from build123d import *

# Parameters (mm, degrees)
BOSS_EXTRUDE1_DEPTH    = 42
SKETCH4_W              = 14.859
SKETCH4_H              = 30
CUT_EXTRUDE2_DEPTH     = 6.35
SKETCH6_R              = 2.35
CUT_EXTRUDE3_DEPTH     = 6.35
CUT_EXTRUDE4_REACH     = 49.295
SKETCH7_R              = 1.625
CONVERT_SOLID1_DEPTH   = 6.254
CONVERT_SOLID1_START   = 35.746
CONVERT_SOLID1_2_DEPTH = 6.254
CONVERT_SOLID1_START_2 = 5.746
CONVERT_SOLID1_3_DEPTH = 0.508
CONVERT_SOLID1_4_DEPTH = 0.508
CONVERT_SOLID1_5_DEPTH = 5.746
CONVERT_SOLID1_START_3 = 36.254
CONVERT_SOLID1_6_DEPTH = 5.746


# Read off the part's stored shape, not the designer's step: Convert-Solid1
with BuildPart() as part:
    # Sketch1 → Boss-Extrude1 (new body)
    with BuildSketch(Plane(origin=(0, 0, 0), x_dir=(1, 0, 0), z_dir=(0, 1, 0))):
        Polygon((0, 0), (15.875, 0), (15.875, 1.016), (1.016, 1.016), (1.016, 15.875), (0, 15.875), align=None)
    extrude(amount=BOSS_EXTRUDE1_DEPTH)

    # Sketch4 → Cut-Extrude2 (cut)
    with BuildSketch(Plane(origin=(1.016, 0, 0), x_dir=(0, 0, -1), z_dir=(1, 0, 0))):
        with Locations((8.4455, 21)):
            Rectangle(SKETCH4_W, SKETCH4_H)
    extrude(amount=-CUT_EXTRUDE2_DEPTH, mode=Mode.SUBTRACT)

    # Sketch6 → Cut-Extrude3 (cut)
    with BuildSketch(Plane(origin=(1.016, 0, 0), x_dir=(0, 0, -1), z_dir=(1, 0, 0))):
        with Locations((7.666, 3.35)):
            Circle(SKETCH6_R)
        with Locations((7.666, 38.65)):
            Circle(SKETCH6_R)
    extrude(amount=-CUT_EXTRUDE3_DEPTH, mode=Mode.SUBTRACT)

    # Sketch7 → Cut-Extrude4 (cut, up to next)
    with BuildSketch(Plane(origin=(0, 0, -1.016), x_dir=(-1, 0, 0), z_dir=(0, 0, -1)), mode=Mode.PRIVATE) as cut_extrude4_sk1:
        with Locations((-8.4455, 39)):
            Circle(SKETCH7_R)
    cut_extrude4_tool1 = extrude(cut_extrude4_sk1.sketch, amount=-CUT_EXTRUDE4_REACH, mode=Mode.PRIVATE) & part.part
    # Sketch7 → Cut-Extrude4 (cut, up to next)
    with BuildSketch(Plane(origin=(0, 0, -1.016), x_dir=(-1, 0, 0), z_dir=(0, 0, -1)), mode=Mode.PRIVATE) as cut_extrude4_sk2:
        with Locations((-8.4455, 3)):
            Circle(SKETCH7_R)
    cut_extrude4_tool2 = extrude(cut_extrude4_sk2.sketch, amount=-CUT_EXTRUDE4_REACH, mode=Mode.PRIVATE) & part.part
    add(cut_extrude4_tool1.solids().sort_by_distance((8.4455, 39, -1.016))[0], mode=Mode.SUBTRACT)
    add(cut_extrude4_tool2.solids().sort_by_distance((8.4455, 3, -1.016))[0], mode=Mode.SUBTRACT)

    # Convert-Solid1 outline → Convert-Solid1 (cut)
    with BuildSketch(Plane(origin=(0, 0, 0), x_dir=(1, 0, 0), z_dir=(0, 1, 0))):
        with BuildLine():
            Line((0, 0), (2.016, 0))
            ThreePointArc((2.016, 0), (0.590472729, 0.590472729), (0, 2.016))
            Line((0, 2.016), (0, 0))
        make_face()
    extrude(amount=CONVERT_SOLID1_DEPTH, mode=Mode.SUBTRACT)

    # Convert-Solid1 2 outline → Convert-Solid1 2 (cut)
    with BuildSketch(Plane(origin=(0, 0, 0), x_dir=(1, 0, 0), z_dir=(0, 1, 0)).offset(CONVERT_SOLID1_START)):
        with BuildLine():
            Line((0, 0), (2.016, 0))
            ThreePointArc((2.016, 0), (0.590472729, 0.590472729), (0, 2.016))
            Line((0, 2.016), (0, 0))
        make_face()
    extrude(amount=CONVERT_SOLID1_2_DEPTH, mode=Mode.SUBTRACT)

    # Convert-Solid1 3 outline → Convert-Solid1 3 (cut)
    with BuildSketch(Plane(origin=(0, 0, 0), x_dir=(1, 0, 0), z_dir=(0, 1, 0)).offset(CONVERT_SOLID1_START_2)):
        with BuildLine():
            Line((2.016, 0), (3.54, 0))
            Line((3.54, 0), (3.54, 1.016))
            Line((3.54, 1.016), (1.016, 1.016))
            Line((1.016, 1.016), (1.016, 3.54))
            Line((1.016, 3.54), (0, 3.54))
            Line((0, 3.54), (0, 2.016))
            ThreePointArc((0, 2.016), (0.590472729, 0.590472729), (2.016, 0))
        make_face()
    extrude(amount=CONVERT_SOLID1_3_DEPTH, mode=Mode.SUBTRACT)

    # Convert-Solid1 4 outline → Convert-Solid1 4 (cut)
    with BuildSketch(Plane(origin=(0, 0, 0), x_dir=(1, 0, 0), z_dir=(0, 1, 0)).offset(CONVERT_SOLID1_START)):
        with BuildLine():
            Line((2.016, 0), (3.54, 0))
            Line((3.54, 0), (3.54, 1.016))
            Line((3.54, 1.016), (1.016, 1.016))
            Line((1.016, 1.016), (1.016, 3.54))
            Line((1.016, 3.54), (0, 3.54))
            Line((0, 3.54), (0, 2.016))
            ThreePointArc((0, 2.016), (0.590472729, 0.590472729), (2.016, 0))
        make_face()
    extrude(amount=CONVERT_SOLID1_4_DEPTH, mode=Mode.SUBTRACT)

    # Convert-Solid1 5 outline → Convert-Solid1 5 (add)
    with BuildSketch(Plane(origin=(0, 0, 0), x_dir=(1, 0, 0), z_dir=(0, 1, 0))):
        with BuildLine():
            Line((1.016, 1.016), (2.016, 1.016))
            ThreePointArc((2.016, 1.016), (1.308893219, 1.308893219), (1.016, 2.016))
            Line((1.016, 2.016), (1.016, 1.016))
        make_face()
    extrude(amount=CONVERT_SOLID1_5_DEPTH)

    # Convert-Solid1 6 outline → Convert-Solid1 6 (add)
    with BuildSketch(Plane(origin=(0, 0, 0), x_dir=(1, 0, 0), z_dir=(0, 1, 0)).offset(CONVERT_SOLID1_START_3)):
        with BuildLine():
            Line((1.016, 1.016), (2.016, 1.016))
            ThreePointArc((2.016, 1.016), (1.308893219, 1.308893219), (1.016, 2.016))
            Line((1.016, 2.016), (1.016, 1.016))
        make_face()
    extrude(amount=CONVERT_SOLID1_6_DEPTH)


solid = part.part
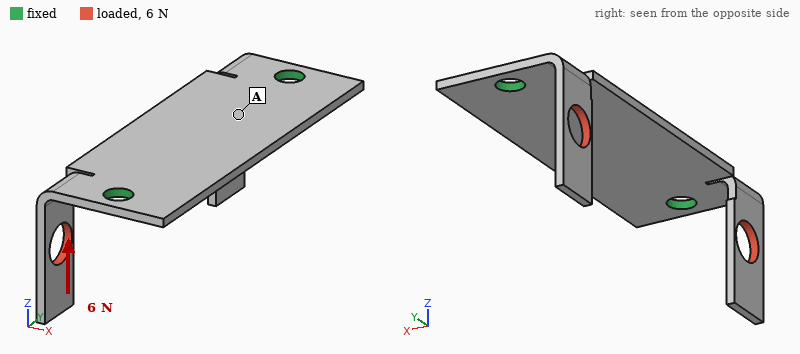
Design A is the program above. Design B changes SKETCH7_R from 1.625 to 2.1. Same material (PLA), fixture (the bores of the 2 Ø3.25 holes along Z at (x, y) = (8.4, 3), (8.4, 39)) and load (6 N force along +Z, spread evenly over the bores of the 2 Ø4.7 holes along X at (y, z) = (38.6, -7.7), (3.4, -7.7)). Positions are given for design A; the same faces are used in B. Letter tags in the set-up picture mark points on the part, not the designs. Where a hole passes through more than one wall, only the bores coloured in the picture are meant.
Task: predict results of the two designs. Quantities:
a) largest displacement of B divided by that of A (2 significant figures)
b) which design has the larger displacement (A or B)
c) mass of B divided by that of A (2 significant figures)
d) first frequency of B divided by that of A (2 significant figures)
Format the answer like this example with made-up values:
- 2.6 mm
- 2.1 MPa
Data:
- 0.87
- A
- 0.99
- 1.0
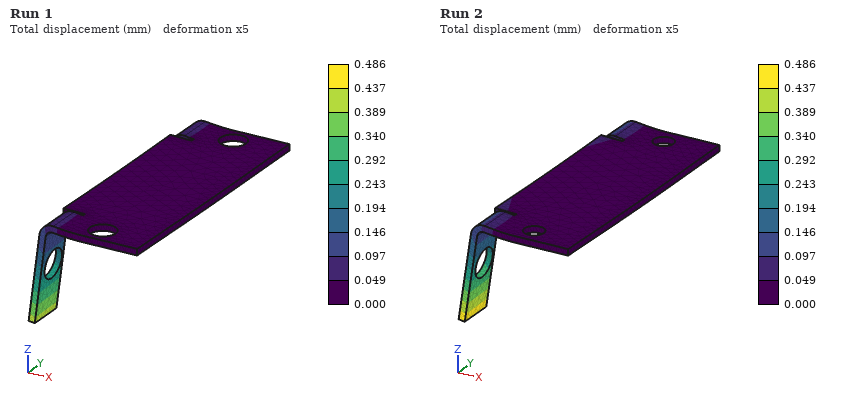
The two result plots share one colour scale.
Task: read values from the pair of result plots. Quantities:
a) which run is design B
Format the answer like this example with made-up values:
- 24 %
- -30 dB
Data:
- Run 1
